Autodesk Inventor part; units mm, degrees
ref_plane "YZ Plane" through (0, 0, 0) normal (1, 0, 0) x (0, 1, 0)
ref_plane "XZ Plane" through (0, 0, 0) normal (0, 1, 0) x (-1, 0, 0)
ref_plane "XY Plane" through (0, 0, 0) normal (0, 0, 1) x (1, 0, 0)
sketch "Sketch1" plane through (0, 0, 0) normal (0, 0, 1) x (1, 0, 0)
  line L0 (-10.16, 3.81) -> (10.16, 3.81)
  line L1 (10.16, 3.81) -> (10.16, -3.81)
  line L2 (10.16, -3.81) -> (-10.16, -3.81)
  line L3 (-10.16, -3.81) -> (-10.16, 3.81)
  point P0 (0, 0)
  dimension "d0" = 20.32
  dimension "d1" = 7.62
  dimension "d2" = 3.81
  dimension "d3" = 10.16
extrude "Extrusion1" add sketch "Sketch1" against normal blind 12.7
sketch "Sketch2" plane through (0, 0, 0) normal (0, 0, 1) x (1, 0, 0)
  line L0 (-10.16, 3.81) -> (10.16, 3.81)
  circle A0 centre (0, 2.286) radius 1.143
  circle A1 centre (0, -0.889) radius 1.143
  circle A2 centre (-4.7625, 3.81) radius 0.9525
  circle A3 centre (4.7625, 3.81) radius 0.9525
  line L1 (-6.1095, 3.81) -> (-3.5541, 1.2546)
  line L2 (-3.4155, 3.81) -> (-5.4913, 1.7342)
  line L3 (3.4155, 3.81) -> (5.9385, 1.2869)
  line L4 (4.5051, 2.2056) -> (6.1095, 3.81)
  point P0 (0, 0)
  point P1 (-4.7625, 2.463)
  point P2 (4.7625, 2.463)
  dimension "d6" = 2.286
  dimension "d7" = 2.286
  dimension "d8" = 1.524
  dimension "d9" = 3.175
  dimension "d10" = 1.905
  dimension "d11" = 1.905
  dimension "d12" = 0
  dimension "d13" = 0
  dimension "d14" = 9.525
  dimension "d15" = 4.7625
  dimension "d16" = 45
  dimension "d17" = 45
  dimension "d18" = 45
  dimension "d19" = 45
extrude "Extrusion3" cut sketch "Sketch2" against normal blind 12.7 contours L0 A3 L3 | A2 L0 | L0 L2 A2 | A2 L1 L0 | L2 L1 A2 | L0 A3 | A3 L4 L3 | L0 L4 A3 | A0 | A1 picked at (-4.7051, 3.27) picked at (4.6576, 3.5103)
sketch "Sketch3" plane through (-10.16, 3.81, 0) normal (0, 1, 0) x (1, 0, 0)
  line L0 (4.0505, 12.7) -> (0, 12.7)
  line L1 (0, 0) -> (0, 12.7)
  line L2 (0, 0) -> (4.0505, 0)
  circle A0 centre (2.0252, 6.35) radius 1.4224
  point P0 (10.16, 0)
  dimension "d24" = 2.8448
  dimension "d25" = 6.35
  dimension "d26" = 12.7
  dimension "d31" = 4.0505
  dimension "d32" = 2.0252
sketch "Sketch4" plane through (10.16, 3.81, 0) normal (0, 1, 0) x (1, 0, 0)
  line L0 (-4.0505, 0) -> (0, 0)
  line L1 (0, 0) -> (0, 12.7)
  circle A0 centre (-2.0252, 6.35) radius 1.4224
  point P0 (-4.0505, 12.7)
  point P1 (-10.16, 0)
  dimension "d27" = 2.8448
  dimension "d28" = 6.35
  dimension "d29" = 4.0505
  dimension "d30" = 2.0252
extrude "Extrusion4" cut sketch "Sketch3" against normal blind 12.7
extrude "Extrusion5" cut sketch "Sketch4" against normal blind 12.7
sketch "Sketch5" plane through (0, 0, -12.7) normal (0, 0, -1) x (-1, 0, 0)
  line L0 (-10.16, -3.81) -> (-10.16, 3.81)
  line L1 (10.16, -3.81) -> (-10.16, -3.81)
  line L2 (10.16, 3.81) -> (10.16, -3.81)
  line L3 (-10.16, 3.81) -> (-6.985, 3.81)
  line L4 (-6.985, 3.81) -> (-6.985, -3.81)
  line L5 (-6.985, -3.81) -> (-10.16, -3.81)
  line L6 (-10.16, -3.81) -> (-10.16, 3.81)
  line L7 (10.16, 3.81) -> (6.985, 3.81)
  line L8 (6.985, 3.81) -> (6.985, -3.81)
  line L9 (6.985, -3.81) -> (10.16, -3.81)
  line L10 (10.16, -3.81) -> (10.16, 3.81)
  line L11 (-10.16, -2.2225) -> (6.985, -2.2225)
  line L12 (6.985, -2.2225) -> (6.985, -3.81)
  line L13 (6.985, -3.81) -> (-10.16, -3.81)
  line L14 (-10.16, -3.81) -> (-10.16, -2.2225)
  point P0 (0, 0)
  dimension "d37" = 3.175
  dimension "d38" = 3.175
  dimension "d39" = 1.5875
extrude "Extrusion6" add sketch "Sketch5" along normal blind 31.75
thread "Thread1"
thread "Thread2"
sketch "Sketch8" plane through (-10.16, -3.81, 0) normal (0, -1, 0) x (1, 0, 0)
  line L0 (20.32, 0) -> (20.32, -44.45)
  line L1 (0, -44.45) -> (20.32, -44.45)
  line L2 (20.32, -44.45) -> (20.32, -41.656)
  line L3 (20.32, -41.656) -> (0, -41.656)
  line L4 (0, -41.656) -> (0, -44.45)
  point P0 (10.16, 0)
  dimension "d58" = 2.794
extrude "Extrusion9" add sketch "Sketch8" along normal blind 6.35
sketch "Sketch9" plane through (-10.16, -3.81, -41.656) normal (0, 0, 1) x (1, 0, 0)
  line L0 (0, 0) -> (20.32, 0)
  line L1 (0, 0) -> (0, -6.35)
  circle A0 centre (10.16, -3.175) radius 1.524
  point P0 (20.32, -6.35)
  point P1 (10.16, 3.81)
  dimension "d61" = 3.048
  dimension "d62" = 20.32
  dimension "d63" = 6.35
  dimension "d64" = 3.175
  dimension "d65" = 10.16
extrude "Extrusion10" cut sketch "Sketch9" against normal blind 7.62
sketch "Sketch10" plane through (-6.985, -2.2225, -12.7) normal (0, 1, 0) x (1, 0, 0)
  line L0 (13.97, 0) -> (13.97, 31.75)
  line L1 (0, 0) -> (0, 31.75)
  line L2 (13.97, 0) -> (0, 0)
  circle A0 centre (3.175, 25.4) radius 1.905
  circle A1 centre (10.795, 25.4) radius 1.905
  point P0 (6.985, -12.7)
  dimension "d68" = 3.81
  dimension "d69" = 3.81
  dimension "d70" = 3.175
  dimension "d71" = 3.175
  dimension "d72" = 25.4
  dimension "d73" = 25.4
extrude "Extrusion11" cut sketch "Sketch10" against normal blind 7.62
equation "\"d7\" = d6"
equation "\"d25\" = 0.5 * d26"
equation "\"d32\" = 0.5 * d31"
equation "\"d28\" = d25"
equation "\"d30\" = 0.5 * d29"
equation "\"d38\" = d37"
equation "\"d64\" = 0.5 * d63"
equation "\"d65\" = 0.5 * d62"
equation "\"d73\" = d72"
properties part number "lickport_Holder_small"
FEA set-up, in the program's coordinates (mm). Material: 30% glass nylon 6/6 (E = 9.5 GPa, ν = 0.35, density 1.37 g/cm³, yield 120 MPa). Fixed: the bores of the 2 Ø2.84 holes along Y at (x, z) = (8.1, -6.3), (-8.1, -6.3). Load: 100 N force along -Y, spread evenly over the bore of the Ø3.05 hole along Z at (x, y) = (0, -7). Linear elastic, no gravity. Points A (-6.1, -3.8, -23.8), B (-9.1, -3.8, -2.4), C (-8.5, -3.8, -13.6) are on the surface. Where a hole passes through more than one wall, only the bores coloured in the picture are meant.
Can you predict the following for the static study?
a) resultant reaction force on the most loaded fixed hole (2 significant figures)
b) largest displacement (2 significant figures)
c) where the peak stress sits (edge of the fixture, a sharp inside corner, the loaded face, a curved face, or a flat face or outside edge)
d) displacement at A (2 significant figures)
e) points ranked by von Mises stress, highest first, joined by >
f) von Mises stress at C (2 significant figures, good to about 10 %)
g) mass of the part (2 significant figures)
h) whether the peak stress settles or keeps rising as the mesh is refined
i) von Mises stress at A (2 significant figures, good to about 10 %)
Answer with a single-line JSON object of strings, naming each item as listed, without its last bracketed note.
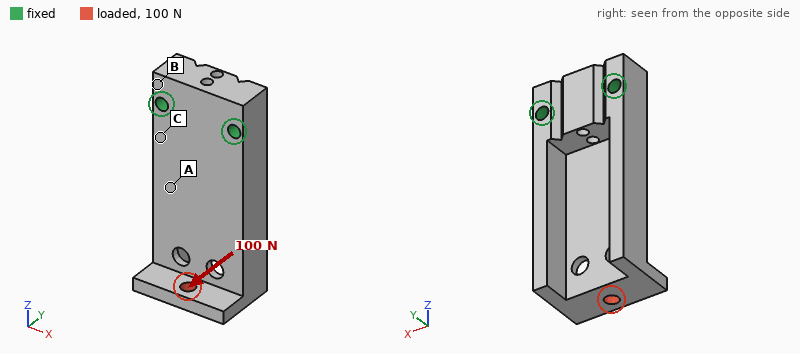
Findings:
{"resultant reaction force on the most loaded fixed hole": "68 N", "largest displacement": "0.51 mm", "where the peak stress sits": "edge of the fixture", "displacement at A": "0.13 mm", "points ranked by von Mises stress, highest first, joined by >": "C > A > B", "von Mises stress at C": "25 MPa", "mass of the part": "5.8 g", "whether the peak stress settles or keeps rising as the mesh is refined": "keeps rising", "von Mises stress at A": "15 MPa"}
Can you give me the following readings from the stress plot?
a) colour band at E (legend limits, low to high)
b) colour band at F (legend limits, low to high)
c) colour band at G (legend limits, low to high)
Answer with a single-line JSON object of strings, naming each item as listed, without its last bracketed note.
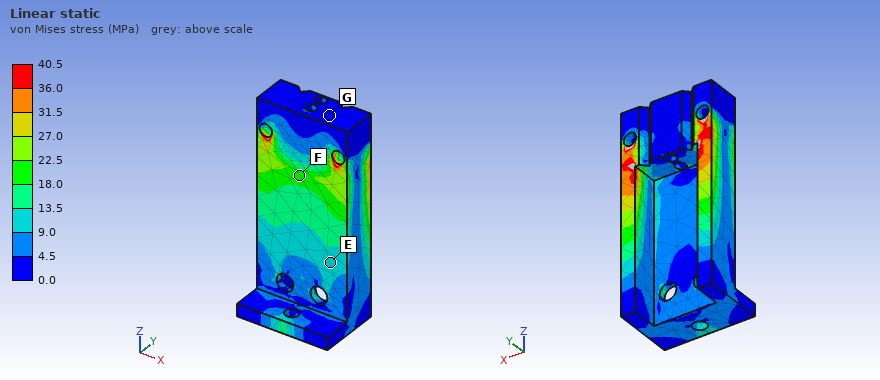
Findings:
{"colour band at E": "9.0 to 13.5 MPa", "colour band at F": "18.0 to 22.5 MPa", "colour band at G": "0.0 to 4.5 MPa"}
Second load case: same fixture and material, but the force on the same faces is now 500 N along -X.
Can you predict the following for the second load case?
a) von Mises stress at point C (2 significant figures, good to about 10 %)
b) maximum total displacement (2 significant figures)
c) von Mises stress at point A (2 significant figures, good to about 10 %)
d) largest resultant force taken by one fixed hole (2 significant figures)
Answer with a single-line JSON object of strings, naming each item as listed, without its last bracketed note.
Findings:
{"von Mises stress at point C": "27 MPa", "maximum total displacement": "0.59 mm", "von Mises stress at point A": "38 MPa", "largest resultant force taken by one fixed hole": "1.1 kN"}
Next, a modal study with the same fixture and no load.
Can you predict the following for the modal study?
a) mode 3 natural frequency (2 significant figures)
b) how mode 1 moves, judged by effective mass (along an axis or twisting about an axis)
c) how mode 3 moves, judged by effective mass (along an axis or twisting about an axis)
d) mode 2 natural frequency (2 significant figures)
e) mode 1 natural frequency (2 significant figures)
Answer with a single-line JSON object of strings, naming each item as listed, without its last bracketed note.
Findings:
{"mode 3 natural frequency": "4900 Hz", "how mode 1 moves, judged by effective mass": "along Y", "how mode 3 moves, judged by effective mass": "along X", "mode 2 natural frequency": "2800 Hz", "mode 1 natural frequency": "2000 Hz"}
